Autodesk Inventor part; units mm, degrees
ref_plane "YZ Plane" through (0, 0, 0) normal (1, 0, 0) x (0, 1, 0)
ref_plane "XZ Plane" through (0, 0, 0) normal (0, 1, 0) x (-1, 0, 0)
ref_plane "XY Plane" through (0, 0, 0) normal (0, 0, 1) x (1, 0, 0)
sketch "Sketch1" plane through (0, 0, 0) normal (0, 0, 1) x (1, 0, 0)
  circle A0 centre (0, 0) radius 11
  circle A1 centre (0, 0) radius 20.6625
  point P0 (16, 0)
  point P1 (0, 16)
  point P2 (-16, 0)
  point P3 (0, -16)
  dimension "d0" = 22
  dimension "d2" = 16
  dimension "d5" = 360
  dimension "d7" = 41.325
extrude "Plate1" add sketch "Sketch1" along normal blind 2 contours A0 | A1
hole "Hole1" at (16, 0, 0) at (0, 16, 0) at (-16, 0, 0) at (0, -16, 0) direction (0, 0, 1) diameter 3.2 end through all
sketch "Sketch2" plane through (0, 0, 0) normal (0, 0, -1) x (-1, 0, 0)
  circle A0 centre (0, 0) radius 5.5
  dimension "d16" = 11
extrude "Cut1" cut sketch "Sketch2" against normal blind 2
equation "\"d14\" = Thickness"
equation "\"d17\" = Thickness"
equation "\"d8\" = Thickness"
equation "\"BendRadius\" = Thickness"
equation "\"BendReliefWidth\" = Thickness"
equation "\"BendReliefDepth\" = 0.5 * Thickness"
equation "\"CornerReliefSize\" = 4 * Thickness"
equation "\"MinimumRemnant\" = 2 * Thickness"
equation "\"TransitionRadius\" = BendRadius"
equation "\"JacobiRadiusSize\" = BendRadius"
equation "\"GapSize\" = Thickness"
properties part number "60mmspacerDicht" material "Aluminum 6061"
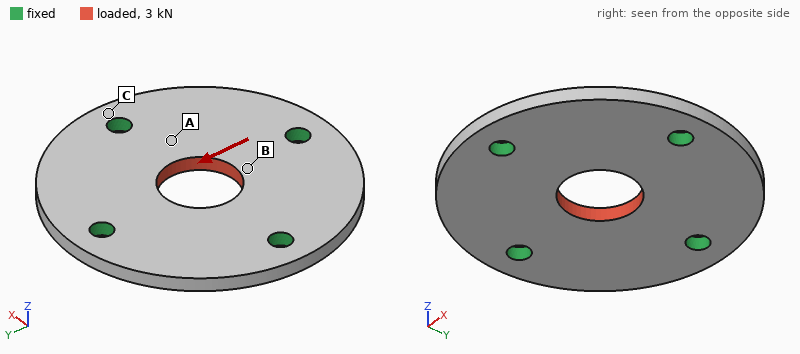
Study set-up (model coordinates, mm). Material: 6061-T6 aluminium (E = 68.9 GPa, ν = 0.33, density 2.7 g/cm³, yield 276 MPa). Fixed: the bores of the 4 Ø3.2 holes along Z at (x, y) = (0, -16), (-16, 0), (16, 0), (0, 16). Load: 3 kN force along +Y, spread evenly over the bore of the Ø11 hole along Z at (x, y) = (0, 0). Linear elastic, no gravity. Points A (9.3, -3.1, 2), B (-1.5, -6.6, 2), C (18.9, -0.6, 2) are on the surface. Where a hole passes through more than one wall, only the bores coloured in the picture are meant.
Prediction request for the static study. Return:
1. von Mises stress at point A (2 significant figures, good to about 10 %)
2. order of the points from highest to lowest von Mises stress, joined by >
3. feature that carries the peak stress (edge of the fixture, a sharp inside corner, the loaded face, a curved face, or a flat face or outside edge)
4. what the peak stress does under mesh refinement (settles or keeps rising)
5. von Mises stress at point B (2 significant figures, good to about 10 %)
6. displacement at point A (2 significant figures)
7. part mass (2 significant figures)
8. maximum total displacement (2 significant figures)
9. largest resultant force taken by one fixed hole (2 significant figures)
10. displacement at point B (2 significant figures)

18 MPa
B > A > C
edge of the fixture
keeps rising
51 MPa
5.0 µm
6.6 g
9.5 µm
940 N
7.0 µm
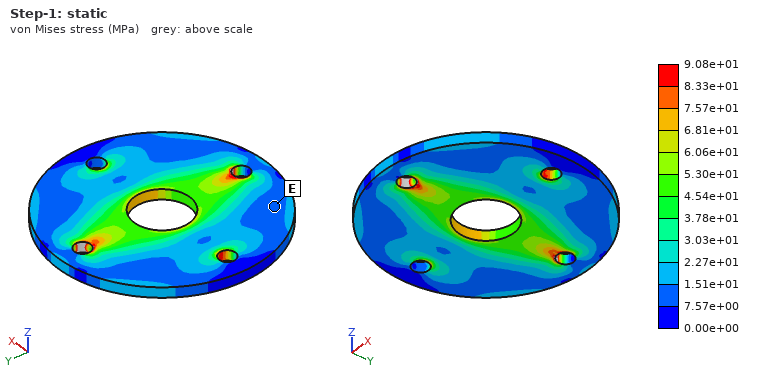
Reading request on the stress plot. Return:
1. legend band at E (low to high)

7.57e+00 to 1.51e+01 MPa
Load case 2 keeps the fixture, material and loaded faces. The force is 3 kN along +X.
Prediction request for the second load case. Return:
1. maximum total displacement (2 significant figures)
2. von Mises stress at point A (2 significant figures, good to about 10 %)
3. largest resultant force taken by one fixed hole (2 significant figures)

9.5 µm
47 MPa
940 N
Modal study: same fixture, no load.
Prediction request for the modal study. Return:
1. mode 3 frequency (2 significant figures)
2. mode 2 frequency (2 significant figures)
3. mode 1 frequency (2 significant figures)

16 kHz
16 kHz
15 kHz
